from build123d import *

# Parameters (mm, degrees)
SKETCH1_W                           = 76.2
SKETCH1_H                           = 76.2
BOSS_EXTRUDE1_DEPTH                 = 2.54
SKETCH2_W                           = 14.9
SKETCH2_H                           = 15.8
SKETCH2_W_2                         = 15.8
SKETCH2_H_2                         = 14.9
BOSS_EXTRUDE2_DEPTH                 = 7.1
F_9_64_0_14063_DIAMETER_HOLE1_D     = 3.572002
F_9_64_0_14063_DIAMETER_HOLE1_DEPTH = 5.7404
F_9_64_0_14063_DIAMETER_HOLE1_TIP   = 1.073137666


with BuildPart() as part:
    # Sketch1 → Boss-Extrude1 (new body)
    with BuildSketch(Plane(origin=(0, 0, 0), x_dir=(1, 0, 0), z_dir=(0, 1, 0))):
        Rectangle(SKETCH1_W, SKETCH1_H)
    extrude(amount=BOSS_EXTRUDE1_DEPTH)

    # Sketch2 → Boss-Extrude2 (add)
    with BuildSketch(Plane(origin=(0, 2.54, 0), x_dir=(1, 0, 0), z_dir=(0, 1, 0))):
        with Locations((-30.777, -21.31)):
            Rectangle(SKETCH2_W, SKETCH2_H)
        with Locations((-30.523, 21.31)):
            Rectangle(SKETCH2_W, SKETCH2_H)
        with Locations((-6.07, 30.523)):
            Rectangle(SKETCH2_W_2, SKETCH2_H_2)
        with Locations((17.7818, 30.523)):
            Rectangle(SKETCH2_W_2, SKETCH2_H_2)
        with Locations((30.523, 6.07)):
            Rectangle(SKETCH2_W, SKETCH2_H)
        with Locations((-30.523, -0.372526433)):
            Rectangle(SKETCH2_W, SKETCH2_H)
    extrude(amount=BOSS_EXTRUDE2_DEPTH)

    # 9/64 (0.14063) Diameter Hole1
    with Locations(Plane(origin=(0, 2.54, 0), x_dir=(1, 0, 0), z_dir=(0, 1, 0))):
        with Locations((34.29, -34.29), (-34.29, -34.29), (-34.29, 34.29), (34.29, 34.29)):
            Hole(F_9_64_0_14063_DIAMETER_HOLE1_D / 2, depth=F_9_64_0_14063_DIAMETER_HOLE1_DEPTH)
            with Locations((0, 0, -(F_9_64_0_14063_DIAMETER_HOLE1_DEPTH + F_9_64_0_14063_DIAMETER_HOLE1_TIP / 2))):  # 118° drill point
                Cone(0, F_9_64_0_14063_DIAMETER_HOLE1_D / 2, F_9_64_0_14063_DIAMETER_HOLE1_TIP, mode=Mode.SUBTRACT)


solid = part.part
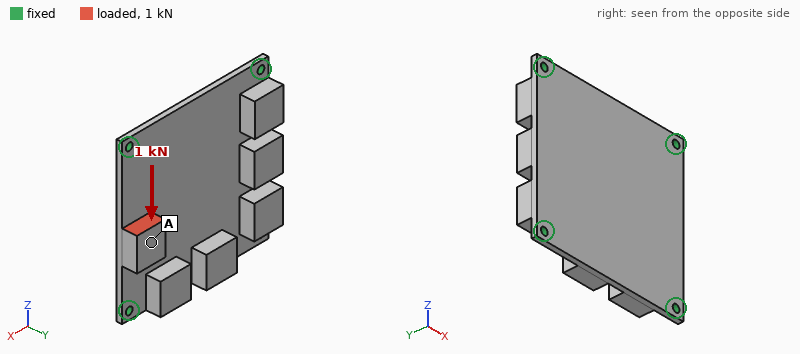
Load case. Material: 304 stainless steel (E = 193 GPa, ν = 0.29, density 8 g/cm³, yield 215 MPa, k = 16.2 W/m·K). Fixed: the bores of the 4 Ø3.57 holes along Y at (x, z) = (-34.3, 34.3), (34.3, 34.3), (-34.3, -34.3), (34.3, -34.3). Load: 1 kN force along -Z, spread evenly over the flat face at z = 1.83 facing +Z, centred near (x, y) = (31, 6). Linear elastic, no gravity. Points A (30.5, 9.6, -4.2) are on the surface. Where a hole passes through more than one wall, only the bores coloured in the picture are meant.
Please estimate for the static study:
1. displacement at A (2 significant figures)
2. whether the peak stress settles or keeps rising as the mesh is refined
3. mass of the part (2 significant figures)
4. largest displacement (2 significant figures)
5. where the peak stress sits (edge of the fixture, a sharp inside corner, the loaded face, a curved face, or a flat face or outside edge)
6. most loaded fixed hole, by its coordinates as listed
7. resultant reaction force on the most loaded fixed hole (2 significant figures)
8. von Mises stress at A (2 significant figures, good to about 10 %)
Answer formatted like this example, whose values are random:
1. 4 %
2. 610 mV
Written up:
1. 20 µm
2. keeps rising
3. 200 g
4. 29 µm
5. edge of the fixture
6. (34.3, -34.3)
7. 470 N
8. 9.5 MPa
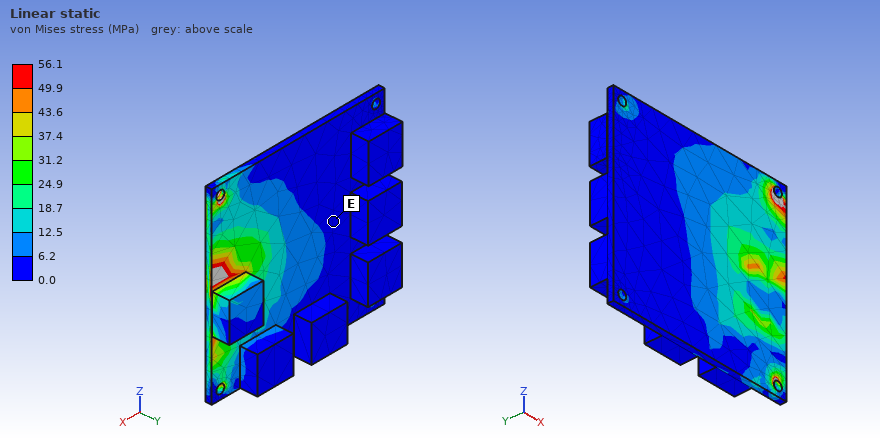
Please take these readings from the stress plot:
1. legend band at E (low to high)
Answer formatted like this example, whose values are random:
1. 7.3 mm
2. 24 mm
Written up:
1. 0.0 to 6.2 MPa
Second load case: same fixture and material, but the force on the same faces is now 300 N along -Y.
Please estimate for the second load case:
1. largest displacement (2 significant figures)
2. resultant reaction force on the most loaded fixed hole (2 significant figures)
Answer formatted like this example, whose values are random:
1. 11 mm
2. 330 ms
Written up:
1. 66 µm
2. 150 N
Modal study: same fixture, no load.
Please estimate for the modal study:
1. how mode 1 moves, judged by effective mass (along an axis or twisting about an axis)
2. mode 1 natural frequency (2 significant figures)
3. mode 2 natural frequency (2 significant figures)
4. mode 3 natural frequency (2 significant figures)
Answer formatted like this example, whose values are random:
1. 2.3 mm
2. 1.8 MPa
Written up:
1. along Y
2. 1600 Hz
3. 2600 Hz
4. 2700 Hz
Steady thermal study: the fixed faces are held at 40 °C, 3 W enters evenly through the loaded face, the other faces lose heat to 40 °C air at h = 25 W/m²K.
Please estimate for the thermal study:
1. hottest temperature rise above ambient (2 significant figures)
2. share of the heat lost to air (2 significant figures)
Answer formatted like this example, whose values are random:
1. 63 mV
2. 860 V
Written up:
1. 33 K
2. 67 %
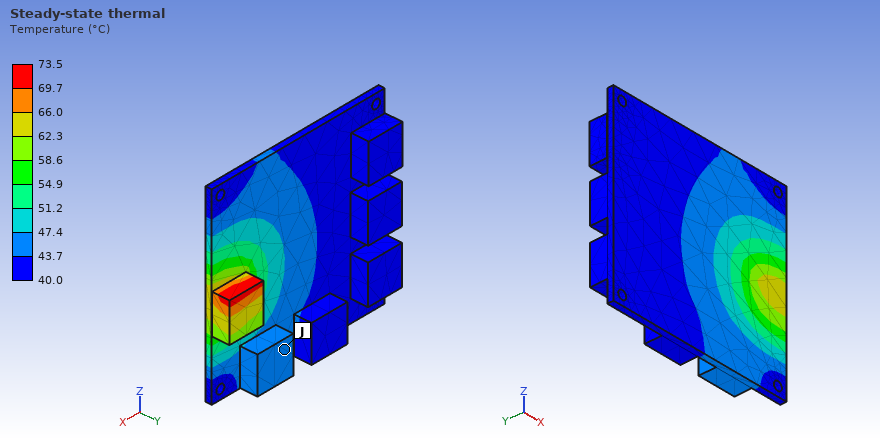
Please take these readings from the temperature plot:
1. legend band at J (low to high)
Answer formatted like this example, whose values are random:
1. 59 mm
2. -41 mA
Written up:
1. 43.7 to 47.4 °C
